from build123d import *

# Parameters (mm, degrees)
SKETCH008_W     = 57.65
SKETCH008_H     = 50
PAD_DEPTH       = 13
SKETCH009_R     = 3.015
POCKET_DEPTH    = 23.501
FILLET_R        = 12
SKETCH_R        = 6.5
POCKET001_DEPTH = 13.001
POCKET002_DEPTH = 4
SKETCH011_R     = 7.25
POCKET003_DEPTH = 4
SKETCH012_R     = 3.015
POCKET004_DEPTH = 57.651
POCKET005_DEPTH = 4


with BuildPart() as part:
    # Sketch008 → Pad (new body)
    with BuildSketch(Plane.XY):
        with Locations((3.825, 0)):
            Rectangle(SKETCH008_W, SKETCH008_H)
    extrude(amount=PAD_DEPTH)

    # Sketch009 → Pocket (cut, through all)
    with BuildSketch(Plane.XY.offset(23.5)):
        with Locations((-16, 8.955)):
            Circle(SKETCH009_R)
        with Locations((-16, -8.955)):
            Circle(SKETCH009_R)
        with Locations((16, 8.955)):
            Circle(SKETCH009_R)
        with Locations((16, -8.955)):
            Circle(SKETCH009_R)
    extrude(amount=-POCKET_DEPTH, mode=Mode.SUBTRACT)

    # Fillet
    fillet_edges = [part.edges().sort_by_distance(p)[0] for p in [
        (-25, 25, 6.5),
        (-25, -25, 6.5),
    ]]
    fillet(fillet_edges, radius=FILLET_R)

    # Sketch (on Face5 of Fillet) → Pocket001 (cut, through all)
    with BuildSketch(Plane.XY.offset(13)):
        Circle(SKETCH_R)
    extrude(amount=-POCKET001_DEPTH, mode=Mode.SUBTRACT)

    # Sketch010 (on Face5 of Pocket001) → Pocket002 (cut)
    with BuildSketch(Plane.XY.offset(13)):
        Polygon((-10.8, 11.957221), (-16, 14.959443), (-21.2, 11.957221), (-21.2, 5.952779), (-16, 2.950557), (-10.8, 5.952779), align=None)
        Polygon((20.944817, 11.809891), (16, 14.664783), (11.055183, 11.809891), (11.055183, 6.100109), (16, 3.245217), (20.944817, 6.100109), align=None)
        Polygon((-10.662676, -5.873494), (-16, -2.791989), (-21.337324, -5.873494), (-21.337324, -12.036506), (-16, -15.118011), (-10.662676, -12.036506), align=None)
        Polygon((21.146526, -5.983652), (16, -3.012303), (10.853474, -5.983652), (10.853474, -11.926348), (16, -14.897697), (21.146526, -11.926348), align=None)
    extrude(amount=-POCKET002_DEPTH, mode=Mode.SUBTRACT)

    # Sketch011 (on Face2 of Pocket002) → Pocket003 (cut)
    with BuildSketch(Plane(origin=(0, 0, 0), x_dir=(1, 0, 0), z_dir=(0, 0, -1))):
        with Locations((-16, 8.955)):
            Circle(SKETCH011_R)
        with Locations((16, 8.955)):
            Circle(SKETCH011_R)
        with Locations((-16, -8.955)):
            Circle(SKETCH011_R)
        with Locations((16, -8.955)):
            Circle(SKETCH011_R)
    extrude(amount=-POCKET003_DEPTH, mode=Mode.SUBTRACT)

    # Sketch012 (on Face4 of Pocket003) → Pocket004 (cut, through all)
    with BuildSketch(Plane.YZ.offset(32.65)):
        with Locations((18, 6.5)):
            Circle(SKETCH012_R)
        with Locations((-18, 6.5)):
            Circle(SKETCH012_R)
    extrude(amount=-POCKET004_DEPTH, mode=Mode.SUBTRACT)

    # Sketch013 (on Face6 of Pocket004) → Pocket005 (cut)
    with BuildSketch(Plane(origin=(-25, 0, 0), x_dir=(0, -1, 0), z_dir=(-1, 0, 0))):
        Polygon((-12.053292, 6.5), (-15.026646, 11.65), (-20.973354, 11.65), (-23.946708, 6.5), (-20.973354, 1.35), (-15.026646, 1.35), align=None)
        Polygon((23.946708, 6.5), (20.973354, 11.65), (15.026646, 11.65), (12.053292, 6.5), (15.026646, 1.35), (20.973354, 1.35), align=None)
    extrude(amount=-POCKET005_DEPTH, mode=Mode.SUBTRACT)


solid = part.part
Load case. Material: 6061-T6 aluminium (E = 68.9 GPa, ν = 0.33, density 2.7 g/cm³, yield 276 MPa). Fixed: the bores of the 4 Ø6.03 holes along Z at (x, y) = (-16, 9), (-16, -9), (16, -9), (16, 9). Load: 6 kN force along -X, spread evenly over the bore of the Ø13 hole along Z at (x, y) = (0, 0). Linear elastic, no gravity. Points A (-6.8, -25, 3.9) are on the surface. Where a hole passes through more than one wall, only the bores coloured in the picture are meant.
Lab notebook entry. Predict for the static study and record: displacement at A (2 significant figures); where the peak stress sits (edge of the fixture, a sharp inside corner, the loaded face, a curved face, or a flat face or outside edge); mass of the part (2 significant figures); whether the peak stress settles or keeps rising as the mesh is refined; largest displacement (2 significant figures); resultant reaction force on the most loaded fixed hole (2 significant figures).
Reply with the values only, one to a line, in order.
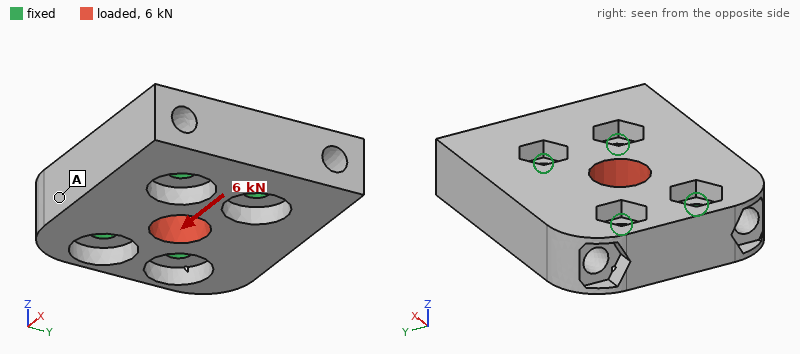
0.85 µm
edge of the fixture
72 g
keeps rising
3.6 µm
1.6 kN
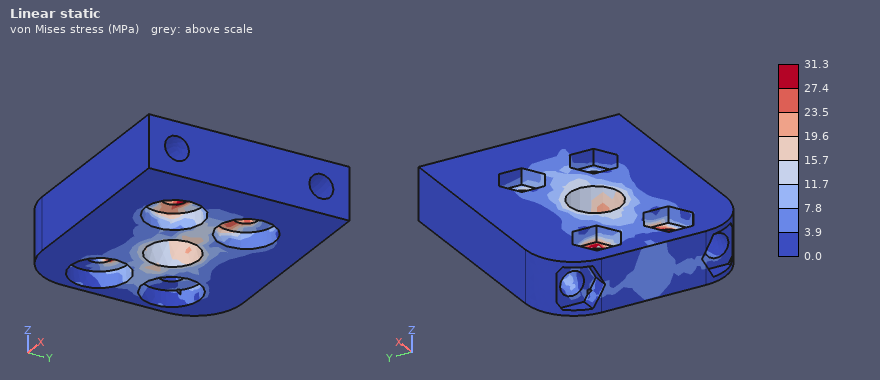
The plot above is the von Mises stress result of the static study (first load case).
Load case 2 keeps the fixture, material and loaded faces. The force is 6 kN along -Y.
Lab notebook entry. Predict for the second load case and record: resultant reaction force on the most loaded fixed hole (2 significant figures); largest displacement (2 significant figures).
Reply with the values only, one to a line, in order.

1.6 kN
5.4 µm
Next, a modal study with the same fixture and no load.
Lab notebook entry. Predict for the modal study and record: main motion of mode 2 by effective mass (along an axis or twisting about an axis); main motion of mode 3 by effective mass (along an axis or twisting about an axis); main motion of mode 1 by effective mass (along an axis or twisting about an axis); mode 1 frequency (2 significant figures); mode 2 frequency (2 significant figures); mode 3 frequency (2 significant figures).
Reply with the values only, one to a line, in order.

along Z
along Z
twisting about X
13 kHz
15 kHz
16 kHz
